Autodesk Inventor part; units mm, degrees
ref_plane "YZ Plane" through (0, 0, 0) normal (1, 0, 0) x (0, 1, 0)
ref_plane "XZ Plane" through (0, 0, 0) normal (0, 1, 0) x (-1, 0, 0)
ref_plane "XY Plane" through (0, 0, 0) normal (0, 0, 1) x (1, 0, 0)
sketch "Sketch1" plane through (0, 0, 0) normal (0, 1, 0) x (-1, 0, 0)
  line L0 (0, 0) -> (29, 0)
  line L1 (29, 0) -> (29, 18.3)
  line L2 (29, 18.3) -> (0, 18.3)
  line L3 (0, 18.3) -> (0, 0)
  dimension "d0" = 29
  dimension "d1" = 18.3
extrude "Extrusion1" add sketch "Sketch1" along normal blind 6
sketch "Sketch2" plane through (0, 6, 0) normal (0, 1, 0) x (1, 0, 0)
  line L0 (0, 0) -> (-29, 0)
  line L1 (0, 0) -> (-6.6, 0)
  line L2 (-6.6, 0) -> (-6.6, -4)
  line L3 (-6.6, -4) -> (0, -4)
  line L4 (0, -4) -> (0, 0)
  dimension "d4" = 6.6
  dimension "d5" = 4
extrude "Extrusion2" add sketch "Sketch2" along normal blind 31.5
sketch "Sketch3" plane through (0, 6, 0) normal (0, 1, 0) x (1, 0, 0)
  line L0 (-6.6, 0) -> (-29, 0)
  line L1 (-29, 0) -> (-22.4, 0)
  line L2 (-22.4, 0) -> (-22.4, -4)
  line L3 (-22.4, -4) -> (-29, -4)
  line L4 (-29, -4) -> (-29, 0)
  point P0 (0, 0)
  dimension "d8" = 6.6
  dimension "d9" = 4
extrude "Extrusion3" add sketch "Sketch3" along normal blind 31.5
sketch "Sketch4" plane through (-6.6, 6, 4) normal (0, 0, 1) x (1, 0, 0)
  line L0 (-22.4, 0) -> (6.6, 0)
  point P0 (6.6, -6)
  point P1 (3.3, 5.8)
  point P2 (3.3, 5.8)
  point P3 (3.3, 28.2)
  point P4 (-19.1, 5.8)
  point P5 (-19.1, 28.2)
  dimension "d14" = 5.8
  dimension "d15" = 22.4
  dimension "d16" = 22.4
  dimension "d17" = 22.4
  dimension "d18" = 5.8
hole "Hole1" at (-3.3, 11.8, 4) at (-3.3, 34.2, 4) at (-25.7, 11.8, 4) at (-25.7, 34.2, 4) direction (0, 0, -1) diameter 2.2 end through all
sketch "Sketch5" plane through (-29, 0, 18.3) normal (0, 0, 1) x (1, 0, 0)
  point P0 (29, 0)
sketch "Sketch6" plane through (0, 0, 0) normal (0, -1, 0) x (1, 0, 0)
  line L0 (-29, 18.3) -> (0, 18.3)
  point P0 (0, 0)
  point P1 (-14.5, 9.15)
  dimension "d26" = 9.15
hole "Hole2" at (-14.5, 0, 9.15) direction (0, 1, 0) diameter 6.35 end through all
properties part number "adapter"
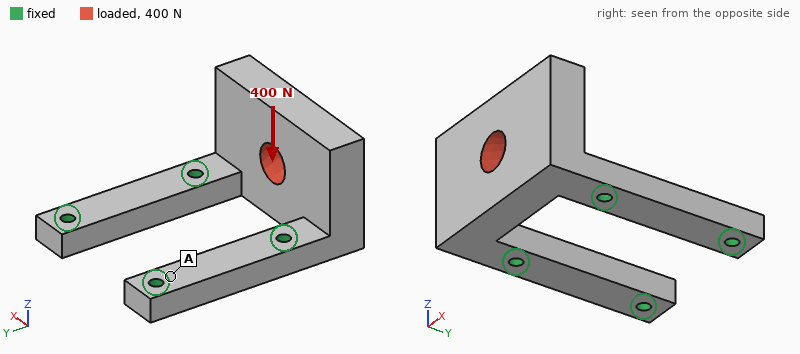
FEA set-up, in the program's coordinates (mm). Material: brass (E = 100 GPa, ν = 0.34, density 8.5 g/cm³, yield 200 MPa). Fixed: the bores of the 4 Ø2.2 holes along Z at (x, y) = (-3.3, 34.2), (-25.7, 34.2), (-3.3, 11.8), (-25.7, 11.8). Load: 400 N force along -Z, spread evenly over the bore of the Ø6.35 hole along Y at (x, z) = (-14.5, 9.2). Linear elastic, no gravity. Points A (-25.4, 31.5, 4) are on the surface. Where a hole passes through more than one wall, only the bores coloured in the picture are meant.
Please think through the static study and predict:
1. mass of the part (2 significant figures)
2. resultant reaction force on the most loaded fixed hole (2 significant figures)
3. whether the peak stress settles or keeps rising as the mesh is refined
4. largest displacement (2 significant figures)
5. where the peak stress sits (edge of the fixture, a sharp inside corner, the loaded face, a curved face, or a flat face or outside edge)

39 g
210 N
keeps rising
39 µm
edge of the fixture
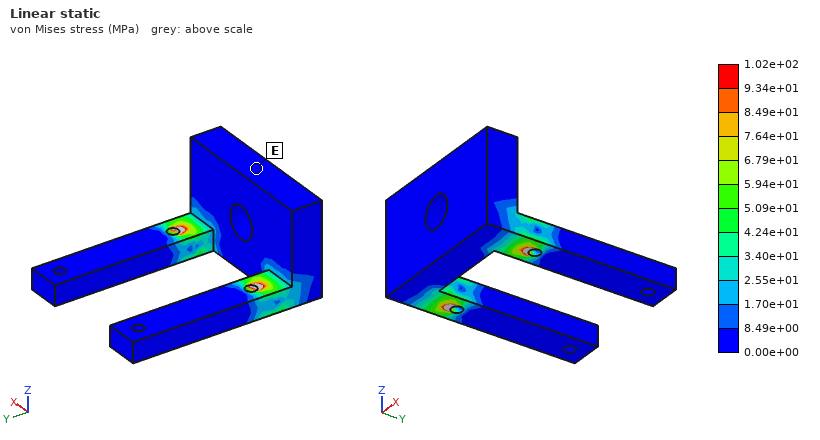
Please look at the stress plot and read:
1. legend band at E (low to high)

0.00e+00 to 8.49e+00 MPa
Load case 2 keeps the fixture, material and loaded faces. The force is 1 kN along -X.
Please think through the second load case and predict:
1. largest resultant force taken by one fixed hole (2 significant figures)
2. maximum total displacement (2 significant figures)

650 N
22 µm
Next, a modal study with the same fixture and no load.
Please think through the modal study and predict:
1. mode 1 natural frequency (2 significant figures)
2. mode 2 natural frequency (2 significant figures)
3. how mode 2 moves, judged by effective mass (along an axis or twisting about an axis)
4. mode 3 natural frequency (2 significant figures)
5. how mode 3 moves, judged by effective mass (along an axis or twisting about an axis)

2900 Hz
7200 Hz
along X
11 kHz
along Z
